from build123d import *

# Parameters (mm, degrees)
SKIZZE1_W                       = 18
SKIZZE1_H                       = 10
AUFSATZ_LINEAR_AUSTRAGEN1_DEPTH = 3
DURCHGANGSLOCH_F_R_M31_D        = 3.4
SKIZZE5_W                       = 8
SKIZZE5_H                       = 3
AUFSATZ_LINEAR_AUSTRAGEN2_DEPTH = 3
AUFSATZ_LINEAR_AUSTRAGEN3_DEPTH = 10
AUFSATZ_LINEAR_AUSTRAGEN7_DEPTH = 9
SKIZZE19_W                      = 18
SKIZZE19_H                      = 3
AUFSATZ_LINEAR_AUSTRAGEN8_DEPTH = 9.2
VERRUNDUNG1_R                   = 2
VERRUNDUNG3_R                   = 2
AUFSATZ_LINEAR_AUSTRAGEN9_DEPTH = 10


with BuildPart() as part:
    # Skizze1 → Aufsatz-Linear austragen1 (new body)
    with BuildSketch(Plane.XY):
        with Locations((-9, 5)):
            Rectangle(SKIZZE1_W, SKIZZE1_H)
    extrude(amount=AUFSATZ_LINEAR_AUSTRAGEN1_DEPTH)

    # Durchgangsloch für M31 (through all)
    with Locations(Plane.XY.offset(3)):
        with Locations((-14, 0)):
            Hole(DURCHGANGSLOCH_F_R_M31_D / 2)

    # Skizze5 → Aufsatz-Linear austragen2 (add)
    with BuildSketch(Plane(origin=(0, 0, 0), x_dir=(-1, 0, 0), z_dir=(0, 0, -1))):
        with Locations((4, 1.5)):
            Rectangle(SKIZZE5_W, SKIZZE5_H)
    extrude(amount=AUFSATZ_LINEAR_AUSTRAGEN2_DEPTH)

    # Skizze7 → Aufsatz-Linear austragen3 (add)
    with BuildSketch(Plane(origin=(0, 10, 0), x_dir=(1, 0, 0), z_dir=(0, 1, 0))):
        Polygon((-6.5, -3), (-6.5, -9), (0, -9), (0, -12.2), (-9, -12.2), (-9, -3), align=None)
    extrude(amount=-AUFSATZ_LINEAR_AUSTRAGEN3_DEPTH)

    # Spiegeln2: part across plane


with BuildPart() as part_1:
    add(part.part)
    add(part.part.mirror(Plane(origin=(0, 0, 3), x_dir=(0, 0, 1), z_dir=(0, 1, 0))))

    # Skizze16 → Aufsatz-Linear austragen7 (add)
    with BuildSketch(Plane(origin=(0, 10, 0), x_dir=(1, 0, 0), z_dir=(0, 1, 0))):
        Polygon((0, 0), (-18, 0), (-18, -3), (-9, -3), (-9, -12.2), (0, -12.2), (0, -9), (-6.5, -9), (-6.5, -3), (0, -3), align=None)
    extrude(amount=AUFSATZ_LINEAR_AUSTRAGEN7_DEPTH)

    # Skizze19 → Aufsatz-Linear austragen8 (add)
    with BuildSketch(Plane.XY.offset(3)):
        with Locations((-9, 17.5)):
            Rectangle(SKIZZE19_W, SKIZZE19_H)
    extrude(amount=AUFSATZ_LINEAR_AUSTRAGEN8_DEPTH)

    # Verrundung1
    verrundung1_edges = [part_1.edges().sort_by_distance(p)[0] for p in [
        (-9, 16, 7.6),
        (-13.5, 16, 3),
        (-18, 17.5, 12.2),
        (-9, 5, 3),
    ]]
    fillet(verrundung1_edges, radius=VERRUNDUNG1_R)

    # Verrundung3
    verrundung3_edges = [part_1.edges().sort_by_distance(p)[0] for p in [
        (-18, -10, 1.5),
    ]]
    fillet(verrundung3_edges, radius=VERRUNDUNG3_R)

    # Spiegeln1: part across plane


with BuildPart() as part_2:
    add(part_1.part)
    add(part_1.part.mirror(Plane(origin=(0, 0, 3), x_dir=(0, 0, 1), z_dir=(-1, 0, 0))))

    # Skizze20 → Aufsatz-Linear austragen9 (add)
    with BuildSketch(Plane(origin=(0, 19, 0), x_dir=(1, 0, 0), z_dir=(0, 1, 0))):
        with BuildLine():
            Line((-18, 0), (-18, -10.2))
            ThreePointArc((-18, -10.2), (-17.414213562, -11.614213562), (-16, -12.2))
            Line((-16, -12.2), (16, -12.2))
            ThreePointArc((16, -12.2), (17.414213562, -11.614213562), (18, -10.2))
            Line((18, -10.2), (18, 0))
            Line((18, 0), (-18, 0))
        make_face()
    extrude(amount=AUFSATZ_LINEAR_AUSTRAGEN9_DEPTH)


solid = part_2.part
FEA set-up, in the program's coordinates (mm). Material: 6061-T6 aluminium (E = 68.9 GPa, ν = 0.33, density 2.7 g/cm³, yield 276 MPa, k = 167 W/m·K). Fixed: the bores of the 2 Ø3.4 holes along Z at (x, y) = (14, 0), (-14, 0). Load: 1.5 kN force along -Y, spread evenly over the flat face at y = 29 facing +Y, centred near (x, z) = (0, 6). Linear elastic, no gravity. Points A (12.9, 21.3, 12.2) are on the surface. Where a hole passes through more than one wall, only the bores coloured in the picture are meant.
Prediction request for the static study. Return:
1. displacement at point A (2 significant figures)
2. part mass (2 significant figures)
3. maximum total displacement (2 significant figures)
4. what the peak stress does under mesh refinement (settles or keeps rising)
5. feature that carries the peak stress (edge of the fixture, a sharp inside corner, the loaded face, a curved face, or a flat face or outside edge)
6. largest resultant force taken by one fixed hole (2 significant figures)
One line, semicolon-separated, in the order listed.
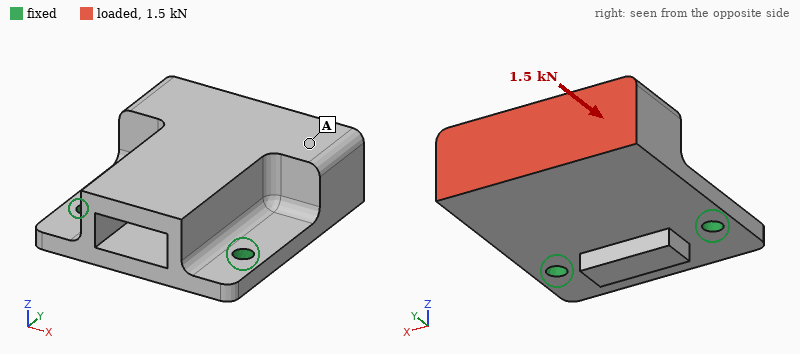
0.087 mm; 30 g; 0.11 mm; keeps rising; edge of the fixture; 750 N
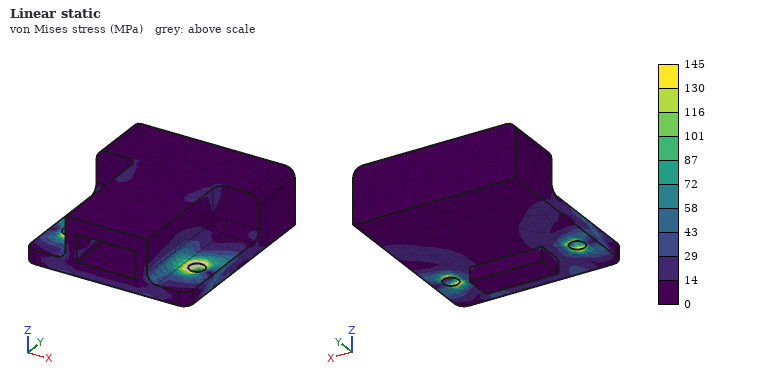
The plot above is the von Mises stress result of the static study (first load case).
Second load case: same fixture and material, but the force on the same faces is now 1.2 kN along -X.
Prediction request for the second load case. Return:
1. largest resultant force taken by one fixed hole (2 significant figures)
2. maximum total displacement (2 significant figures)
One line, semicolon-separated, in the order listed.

1.4 kN; 26 µm
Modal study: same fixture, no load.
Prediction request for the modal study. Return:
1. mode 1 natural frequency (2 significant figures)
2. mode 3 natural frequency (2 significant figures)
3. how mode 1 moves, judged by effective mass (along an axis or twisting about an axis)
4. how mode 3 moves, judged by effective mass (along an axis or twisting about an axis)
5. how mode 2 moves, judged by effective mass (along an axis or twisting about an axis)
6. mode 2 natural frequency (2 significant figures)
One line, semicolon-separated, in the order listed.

2200 Hz; 11 kHz; along Z; along X; along X; 8500 Hz
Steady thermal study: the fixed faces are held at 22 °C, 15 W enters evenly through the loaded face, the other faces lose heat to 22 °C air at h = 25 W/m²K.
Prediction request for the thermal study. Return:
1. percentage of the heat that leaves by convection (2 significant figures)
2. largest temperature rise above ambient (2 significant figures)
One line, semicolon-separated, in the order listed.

6.5 %; 14 K
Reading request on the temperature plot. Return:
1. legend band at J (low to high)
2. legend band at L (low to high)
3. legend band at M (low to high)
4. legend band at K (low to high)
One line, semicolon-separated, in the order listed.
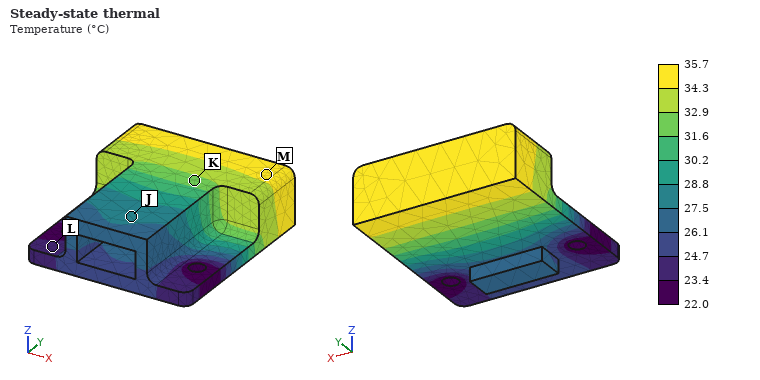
27.5 to 28.8 °C; 23.4 to 24.7 °C; 34.3 to 35.7 °C; 31.6 to 32.9 °C
